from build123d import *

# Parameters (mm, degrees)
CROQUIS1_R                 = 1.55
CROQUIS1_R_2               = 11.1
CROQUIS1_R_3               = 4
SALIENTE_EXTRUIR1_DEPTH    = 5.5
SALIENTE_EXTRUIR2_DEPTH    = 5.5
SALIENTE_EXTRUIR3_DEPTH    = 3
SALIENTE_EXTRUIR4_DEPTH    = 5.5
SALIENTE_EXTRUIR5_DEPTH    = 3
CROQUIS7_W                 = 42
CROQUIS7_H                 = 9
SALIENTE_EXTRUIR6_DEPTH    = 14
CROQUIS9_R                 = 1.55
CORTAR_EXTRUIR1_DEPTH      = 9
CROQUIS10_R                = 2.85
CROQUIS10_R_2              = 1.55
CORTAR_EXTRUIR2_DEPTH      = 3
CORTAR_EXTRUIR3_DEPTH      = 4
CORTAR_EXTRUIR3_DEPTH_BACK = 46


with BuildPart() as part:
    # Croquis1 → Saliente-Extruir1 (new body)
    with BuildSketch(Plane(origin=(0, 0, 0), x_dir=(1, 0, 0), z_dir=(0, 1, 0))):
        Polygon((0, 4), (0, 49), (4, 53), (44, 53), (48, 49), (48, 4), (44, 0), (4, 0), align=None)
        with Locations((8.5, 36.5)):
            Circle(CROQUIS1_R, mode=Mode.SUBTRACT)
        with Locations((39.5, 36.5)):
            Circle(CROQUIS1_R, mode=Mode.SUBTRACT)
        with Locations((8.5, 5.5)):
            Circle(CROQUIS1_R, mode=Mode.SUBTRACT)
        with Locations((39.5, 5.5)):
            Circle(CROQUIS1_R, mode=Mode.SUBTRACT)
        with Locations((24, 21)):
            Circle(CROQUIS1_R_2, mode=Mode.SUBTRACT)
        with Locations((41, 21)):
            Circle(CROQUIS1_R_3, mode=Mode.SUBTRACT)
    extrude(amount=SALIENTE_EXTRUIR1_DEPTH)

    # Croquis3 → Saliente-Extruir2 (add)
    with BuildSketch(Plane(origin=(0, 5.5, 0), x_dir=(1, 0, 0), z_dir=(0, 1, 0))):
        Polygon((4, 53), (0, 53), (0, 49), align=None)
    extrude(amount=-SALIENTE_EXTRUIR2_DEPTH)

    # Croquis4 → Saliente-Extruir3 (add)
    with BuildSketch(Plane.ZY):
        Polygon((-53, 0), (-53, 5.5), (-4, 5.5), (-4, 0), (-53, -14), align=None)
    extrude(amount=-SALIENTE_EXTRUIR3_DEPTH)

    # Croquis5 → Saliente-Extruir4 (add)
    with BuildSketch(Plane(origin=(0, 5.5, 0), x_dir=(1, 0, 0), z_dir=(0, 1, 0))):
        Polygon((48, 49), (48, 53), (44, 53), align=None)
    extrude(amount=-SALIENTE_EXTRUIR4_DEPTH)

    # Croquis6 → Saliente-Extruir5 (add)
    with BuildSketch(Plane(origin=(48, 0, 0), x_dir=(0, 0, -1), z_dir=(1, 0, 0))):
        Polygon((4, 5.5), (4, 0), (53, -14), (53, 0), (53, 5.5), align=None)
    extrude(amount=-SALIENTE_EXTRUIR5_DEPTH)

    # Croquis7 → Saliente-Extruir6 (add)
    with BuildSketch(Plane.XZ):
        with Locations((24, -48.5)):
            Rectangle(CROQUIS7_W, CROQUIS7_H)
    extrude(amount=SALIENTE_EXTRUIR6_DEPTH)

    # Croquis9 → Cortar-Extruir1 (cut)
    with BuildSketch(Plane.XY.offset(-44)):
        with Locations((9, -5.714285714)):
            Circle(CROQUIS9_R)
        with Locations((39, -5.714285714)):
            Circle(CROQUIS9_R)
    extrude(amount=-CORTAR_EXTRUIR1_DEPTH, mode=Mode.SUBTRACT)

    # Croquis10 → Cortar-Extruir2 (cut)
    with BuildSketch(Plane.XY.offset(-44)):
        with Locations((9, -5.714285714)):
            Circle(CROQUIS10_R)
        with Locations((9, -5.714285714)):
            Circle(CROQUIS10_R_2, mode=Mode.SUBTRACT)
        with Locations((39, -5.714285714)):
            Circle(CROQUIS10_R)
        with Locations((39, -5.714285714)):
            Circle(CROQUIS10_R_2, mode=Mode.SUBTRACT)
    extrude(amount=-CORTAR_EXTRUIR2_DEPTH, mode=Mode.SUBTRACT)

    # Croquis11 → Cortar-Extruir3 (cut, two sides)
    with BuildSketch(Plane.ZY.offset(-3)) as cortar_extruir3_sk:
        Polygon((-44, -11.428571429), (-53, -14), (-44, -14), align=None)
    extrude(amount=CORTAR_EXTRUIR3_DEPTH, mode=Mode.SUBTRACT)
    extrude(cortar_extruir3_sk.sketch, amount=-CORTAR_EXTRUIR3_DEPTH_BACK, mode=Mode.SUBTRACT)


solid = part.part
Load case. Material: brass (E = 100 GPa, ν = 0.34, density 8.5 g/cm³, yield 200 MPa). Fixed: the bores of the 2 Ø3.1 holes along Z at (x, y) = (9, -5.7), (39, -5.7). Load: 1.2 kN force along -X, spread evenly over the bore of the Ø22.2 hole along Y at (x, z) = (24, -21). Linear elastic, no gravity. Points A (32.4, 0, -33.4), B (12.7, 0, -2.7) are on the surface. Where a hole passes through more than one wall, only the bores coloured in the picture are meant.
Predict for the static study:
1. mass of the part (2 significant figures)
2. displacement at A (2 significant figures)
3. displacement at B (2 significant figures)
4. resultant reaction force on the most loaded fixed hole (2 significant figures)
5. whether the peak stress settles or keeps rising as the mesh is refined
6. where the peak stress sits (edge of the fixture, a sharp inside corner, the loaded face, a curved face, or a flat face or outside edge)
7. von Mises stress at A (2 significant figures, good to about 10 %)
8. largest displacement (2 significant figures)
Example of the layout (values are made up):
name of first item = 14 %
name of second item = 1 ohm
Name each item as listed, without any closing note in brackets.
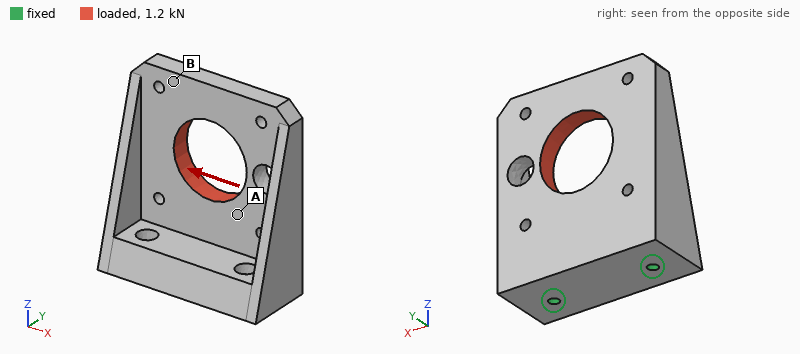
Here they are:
mass of the part = 150 g
displacement at A = 8.9 µm
displacement at B = 33 µm
resultant reaction force on the most loaded fixed hole = 1.2 kN
whether the peak stress settles or keeps rising as the mesh is refined = keeps rising
where the peak stress sits = edge of the fixture
von Mises stress at A = 15 MPa
largest displacement = 38 µm
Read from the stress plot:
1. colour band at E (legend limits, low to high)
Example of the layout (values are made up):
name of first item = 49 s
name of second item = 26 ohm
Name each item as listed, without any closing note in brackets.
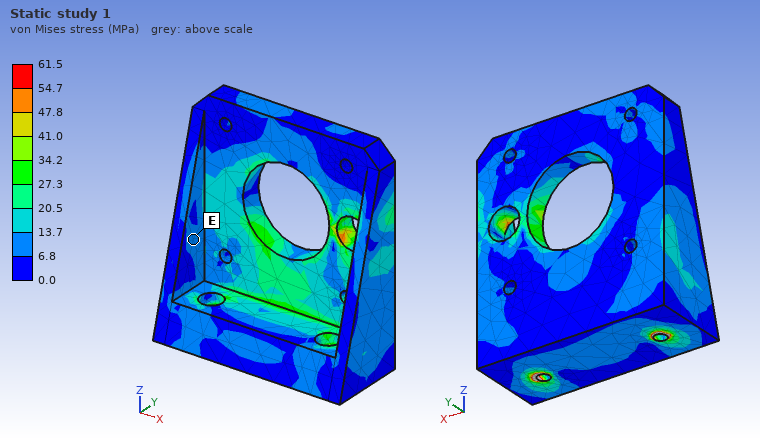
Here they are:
colour band at E = 6.8 to 13.7 MPa
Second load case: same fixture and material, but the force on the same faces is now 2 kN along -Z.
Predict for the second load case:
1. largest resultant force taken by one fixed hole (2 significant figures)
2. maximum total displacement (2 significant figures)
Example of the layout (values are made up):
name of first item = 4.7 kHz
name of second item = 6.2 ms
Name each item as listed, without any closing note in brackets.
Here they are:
largest resultant force taken by one fixed hole = 1.0 kN
maximum total displacement = 57 µm
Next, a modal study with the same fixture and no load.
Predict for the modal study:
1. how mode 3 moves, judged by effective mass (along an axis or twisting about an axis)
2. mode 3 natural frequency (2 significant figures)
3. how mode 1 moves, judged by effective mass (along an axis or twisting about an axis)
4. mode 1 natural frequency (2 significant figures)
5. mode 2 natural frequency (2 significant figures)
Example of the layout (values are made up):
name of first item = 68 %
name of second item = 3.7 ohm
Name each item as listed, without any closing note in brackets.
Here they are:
how mode 3 moves, judged by effective mass = along X
mode 3 natural frequency = 5100 Hz
how mode 1 moves, judged by effective mass = along Y
mode 1 natural frequency = 1700 Hz
mode 2 natural frequency = 3000 Hz
